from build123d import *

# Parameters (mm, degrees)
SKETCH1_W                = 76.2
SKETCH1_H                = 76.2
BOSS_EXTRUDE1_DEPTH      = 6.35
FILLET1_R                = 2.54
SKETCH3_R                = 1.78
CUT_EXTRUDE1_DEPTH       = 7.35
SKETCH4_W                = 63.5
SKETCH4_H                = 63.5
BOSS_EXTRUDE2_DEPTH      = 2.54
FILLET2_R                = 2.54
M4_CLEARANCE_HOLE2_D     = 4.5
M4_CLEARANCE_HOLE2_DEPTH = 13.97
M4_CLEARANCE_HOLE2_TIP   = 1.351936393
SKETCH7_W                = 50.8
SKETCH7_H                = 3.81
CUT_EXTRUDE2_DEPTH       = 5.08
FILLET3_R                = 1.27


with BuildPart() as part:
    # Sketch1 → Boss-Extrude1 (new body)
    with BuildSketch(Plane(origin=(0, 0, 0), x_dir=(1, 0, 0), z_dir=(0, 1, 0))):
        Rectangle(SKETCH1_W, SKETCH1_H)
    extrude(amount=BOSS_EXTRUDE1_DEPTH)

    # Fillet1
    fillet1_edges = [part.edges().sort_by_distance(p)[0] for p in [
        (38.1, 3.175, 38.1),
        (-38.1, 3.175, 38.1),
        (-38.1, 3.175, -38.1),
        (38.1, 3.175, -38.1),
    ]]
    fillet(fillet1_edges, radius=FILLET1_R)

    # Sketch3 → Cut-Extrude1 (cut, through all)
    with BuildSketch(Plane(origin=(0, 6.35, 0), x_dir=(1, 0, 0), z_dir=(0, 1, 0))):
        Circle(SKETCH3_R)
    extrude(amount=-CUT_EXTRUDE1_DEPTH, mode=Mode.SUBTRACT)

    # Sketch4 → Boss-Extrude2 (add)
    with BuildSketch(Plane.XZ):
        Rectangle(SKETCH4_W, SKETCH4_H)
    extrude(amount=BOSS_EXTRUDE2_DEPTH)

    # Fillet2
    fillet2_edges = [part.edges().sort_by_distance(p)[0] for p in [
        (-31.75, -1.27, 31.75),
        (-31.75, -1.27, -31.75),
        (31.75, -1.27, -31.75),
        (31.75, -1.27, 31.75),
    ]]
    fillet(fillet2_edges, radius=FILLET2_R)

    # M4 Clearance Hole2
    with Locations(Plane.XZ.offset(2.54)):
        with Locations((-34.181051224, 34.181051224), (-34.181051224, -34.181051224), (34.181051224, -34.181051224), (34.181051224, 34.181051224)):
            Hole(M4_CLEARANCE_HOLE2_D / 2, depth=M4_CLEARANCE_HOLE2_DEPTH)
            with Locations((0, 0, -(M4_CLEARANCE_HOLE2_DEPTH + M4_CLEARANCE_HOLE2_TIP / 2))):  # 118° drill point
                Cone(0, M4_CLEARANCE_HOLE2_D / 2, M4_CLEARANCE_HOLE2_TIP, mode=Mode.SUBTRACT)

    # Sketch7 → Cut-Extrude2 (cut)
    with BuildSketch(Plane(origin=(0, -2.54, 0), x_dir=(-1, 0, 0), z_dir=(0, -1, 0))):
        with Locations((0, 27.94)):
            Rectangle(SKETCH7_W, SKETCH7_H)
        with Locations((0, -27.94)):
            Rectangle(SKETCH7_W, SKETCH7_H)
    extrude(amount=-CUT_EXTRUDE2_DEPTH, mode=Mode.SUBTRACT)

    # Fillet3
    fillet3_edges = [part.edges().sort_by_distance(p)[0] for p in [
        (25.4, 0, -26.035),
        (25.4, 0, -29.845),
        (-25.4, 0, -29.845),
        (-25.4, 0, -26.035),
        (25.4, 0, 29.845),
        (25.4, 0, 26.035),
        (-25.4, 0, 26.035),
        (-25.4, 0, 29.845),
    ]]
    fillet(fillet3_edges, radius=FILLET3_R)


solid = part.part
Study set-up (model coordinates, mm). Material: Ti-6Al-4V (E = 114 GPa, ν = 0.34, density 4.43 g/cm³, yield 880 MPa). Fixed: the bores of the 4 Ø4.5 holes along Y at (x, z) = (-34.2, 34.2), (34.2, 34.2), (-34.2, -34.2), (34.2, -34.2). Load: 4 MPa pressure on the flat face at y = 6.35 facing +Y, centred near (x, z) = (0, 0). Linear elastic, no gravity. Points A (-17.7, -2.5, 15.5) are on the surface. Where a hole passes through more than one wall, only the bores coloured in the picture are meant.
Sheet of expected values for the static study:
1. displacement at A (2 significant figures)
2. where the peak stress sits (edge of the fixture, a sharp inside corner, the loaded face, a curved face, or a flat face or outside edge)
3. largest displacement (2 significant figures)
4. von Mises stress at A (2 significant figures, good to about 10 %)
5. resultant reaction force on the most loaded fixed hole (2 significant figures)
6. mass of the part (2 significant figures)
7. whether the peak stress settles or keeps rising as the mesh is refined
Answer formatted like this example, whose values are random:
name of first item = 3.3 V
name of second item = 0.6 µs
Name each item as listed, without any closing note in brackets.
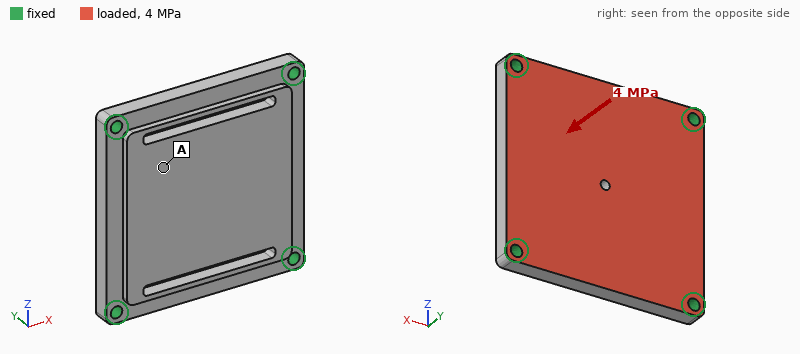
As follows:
displacement at A = 0.13 mm
where the peak stress sits = edge of the fixture
largest displacement = 0.17 mm
von Mises stress at A = 100 MPa
resultant reaction force on the most loaded fixed hole = 6.2 kN
mass of the part = 200 g
whether the peak stress settles or keeps rising as the mesh is refined = keeps rising
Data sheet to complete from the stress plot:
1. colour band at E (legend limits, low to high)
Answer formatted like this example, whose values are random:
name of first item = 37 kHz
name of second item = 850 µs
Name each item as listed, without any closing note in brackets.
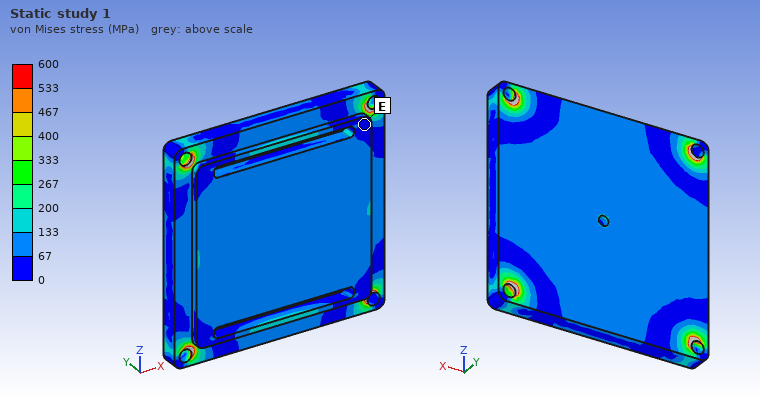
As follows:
colour band at E = 0 to 67 MPa
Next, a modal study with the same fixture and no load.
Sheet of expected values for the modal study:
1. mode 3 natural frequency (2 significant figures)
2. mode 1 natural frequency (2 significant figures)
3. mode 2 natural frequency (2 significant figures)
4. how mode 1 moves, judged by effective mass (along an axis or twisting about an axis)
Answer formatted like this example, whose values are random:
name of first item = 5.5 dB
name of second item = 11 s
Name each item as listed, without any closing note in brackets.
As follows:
mode 3 natural frequency = 8200 Hz
mode 1 natural frequency = 4700 Hz
mode 2 natural frequency = 8100 Hz
how mode 1 moves, judged by effective mass = along Y
